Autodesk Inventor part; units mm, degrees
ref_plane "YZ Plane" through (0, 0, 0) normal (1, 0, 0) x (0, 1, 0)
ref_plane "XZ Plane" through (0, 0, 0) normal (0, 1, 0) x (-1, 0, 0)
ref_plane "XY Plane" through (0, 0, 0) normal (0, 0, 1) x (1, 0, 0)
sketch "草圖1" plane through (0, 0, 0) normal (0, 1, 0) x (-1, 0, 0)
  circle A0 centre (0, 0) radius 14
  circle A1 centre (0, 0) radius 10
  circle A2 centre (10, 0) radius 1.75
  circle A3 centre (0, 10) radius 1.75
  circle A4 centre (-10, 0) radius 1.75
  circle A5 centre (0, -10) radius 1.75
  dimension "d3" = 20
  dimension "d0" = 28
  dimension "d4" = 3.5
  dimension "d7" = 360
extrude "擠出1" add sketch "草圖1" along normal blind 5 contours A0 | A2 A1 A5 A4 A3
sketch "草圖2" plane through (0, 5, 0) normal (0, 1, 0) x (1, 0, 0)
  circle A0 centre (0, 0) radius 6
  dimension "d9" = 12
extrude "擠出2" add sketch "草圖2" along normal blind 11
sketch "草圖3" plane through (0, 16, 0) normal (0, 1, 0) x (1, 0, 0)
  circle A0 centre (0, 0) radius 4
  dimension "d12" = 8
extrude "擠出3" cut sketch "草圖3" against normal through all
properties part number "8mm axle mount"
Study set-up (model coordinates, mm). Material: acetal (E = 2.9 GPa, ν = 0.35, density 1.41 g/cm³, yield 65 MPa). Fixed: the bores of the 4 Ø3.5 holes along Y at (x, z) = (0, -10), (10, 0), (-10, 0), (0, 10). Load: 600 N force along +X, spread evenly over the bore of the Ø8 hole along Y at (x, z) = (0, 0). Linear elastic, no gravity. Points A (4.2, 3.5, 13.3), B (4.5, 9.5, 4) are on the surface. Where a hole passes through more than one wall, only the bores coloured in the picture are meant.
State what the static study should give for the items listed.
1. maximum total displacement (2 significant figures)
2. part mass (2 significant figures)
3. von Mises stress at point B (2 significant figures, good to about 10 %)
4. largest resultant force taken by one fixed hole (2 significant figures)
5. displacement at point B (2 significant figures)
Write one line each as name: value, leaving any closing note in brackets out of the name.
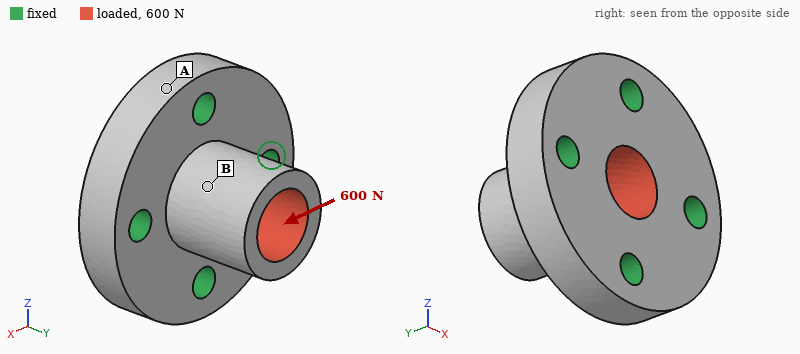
maximum total displacement: 0.15 mm
part mass: 4.7 g
von Mises stress at point B: 7.5 MPa
largest resultant force taken by one fixed hole: 260 N
displacement at point B: 0.082 mm
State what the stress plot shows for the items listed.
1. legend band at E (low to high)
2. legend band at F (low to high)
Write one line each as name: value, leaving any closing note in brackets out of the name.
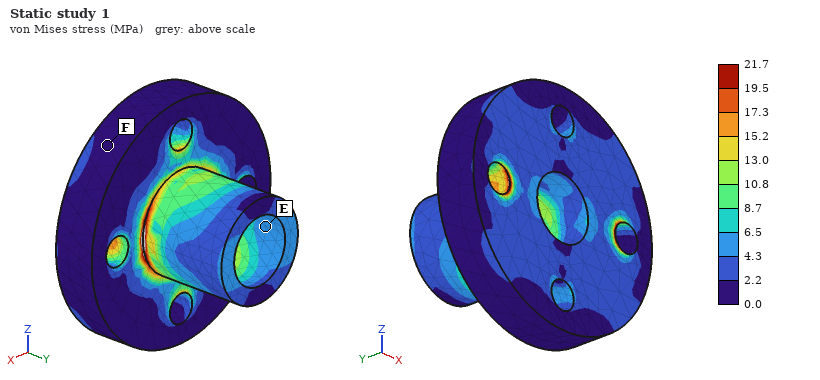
legend band at E: 4.3 to 6.5 MPa
legend band at F: 0.0 to 2.2 MPa
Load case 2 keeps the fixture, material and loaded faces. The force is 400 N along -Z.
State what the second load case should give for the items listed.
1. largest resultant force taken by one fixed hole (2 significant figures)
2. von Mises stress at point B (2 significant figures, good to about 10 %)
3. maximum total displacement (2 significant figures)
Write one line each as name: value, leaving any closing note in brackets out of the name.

largest resultant force taken by one fixed hole: 180 N
von Mises stress at point B: 5.4 MPa
maximum total displacement: 0.10 mm
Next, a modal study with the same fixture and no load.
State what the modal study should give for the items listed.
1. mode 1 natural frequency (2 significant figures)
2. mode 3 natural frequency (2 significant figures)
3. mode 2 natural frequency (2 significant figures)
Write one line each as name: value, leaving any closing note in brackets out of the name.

mode 1 natural frequency: 9800 Hz
mode 3 natural frequency: 16 kHz
mode 2 natural frequency: 9800 Hz
